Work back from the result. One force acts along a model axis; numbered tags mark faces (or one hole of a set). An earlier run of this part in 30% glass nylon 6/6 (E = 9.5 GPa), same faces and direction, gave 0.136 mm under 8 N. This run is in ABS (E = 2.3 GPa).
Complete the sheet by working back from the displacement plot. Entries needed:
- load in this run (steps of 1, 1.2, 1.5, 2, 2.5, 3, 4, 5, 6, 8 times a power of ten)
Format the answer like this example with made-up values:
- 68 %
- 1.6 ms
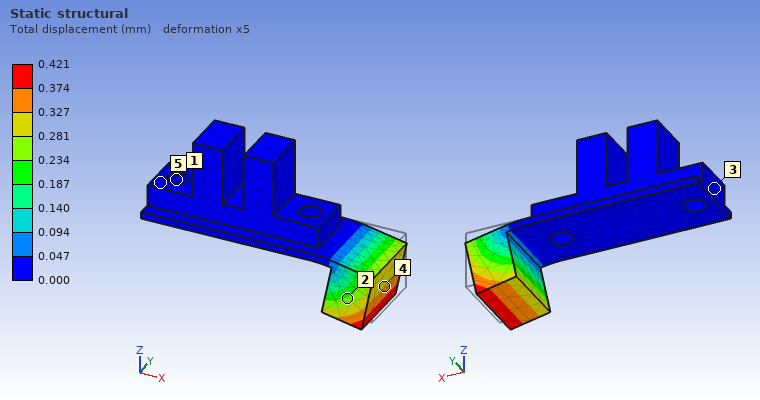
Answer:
- 6 N
